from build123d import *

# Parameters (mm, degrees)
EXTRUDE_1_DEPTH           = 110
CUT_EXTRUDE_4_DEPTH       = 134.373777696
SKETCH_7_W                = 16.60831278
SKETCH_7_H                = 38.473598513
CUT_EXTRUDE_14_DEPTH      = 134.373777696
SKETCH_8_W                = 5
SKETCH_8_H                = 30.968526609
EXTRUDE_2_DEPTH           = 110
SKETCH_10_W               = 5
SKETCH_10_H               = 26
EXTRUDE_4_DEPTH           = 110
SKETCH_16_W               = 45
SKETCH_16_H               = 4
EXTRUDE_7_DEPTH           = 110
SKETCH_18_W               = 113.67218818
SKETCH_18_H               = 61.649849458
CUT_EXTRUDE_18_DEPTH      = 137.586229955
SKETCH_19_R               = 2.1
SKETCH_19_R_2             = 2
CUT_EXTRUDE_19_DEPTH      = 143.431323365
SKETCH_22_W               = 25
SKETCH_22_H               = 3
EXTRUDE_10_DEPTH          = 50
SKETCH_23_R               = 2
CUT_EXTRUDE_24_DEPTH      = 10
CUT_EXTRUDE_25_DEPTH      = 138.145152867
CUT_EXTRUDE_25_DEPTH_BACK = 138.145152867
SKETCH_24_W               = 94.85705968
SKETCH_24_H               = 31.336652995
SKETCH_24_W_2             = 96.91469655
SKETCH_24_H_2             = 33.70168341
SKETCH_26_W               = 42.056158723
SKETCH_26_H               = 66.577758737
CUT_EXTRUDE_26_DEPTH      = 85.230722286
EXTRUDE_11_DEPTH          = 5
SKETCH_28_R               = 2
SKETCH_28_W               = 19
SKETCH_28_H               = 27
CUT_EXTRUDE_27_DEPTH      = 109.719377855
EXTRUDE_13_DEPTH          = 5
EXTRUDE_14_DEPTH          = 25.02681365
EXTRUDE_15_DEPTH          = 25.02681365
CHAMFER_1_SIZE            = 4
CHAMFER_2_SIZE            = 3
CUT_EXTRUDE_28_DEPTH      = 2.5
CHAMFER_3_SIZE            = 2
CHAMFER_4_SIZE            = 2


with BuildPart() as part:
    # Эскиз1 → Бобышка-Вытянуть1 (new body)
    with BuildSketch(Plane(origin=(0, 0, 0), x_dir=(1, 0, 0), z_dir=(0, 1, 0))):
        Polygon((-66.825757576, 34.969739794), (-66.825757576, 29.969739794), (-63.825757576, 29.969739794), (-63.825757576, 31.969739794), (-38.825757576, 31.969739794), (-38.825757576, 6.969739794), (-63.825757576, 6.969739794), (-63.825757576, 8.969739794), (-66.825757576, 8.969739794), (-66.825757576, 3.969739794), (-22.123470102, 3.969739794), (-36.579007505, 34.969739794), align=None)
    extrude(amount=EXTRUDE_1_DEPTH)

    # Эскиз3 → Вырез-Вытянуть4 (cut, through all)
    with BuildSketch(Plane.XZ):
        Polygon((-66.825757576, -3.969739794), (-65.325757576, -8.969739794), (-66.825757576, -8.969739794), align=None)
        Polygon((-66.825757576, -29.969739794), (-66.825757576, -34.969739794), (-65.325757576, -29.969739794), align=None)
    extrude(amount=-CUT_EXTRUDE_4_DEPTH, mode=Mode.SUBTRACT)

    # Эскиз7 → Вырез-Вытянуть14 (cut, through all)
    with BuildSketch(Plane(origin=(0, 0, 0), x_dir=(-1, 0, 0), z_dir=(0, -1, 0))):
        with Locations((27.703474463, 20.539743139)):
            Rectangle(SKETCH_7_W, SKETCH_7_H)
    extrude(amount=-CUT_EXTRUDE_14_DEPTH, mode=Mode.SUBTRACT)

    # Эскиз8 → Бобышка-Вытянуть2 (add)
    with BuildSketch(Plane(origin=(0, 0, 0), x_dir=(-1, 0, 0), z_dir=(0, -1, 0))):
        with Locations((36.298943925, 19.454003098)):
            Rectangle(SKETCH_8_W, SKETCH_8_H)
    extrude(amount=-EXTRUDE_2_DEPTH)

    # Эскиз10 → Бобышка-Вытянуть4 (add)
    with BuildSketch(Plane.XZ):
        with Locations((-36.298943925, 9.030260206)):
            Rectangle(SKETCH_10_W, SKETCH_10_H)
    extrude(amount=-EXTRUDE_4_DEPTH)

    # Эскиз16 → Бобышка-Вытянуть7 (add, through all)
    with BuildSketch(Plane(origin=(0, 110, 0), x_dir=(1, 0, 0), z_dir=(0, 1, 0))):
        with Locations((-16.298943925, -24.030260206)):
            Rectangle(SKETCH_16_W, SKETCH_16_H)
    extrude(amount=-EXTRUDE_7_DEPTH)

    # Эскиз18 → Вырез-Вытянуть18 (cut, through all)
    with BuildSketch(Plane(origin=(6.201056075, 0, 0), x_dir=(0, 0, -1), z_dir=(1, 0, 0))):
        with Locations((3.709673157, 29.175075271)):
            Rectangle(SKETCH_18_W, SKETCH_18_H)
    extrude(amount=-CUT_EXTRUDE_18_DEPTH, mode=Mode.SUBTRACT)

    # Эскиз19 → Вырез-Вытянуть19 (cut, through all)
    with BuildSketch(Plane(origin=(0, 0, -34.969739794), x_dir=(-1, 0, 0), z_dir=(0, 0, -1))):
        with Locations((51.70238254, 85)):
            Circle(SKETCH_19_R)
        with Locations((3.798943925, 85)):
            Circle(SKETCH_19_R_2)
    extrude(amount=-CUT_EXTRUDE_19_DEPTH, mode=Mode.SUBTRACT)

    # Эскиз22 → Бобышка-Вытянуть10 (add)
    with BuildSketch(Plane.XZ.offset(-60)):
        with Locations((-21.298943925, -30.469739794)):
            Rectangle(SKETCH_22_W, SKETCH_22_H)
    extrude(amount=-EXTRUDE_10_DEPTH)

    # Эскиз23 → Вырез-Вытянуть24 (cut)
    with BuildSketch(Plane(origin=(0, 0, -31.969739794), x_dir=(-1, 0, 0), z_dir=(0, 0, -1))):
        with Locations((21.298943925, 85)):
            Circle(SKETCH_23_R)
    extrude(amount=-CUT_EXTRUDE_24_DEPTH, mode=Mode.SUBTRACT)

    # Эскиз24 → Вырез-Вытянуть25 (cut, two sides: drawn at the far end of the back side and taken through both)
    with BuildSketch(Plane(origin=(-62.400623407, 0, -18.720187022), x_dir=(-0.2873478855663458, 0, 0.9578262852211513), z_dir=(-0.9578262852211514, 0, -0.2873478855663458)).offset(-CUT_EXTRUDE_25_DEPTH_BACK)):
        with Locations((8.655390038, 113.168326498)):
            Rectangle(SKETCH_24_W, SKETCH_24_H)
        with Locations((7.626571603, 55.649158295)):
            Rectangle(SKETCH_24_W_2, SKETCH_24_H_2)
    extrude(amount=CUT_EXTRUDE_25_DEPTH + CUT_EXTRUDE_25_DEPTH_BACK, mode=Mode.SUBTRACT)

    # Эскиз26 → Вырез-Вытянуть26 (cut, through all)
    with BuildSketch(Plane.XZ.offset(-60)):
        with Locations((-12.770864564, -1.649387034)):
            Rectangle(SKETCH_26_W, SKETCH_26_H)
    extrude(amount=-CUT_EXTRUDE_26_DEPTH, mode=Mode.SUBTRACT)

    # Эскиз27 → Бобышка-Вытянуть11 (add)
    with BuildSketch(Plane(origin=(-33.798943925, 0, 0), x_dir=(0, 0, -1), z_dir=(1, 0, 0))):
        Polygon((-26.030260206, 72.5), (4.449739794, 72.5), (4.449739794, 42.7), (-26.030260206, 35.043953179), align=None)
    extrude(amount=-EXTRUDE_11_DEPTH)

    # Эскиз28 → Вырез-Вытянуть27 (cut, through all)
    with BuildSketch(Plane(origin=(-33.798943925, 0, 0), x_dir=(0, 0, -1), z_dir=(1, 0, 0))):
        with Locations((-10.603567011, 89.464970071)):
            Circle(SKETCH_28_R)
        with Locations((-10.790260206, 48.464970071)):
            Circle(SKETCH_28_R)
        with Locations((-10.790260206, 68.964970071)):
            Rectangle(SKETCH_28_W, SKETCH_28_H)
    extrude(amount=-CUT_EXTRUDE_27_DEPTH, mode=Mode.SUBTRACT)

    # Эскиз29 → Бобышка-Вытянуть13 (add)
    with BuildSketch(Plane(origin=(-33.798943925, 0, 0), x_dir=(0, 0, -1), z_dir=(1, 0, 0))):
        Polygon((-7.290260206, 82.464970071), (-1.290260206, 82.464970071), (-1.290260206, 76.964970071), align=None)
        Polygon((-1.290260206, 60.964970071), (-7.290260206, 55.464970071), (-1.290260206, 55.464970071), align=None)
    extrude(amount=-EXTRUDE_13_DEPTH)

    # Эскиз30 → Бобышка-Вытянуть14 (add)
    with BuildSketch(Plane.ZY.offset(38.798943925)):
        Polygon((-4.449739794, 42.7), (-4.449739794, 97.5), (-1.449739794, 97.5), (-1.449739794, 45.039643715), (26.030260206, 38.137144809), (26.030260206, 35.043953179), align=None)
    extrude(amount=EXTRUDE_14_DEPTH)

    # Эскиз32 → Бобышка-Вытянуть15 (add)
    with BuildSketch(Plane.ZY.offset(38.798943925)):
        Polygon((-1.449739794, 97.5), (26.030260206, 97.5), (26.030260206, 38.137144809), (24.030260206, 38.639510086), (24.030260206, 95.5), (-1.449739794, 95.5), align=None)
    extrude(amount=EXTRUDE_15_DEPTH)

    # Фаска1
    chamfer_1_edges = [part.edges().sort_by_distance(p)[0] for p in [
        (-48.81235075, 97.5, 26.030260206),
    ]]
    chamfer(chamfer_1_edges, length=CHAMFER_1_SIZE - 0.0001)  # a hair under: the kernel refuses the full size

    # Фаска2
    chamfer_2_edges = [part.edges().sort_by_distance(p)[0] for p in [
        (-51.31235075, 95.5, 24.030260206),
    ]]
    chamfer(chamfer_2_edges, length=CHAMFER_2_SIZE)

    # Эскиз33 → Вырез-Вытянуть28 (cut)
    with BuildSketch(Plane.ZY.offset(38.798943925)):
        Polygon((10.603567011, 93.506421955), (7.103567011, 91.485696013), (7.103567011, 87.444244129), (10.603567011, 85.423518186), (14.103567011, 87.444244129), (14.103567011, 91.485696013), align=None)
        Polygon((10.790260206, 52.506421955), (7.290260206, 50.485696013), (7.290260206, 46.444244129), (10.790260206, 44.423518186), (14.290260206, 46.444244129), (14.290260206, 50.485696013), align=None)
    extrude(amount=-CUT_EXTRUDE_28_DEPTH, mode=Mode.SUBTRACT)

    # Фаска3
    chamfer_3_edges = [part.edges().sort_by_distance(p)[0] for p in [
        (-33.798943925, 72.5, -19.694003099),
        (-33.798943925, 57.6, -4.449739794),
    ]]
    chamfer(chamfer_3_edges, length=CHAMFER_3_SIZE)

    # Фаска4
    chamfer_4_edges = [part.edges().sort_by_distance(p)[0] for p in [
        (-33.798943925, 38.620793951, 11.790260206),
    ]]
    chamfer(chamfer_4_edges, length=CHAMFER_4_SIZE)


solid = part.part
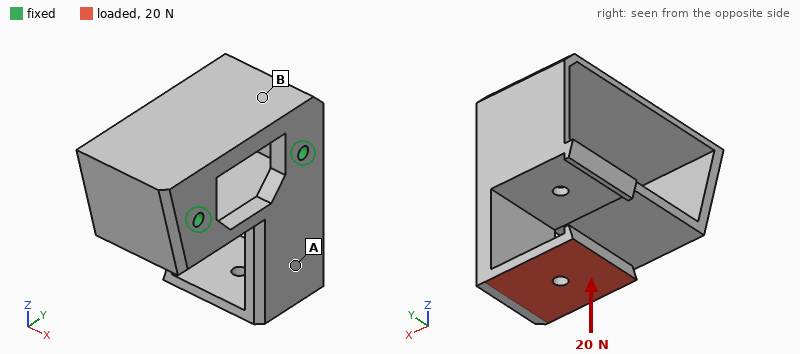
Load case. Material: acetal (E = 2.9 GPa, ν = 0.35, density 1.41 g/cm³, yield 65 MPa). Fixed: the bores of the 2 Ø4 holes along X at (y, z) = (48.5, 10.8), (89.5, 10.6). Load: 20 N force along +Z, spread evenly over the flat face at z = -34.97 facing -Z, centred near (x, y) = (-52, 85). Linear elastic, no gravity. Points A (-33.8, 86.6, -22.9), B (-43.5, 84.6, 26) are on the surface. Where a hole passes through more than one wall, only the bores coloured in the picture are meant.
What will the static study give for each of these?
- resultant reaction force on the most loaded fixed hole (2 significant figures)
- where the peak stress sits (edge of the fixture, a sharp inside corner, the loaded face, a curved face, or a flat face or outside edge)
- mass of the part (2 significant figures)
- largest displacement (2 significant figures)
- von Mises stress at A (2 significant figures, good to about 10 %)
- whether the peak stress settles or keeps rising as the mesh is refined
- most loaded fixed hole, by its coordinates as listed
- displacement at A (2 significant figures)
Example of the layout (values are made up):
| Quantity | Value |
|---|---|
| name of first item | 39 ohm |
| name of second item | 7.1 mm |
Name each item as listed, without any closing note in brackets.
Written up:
| Quantity | Value |
|---|---|
| resultant reaction force on the most loaded fixed hole | 18 N |
| where the peak stress sits | edge of the fixture |
| mass of the part | 34 g |
| largest displacement | 0.93 mm |
| von Mises stress at A | 2.5 MPa |
| whether the peak stress settles or keeps rising as the mesh is refined | keeps rising |
| most loaded fixed hole, by its coordinates as listed | (89.5, 10.6) |
| displacement at A | 0.20 mm |
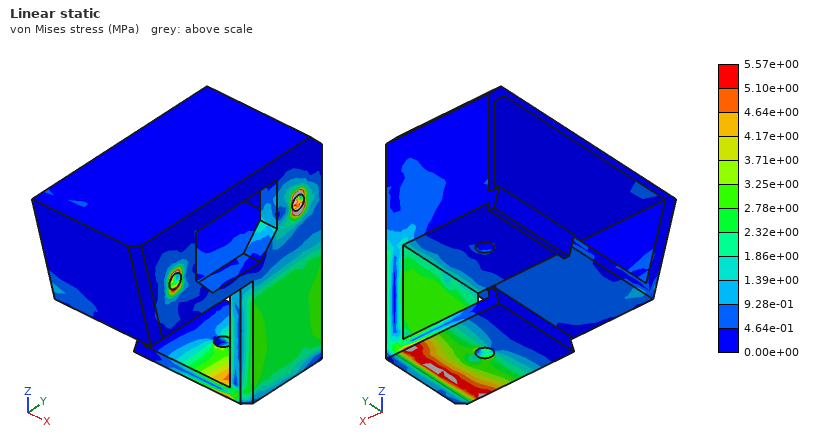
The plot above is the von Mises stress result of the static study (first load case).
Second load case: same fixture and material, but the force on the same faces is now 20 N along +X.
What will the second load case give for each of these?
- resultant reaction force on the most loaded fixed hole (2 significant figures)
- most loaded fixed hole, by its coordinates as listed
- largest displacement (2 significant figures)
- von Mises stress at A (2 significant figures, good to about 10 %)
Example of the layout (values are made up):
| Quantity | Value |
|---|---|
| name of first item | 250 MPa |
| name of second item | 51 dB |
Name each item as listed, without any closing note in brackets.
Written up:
| Quantity | Value |
|---|---|
| resultant reaction force on the most loaded fixed hole | 17 N |
| most loaded fixed hole, by its coordinates as listed | (89.5, 10.6) |
| largest displacement | 1.1 mm |
| von Mises stress at A | 2.2 MPa |
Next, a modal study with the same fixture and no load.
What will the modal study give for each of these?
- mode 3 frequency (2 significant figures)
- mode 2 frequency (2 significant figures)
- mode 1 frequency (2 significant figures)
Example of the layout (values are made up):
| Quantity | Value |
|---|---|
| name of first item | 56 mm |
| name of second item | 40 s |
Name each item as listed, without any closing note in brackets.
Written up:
| Quantity | Value |
|---|---|
| mode 3 frequency | 760 Hz |
| mode 2 frequency | 650 Hz |
| mode 1 frequency | 310 Hz |
